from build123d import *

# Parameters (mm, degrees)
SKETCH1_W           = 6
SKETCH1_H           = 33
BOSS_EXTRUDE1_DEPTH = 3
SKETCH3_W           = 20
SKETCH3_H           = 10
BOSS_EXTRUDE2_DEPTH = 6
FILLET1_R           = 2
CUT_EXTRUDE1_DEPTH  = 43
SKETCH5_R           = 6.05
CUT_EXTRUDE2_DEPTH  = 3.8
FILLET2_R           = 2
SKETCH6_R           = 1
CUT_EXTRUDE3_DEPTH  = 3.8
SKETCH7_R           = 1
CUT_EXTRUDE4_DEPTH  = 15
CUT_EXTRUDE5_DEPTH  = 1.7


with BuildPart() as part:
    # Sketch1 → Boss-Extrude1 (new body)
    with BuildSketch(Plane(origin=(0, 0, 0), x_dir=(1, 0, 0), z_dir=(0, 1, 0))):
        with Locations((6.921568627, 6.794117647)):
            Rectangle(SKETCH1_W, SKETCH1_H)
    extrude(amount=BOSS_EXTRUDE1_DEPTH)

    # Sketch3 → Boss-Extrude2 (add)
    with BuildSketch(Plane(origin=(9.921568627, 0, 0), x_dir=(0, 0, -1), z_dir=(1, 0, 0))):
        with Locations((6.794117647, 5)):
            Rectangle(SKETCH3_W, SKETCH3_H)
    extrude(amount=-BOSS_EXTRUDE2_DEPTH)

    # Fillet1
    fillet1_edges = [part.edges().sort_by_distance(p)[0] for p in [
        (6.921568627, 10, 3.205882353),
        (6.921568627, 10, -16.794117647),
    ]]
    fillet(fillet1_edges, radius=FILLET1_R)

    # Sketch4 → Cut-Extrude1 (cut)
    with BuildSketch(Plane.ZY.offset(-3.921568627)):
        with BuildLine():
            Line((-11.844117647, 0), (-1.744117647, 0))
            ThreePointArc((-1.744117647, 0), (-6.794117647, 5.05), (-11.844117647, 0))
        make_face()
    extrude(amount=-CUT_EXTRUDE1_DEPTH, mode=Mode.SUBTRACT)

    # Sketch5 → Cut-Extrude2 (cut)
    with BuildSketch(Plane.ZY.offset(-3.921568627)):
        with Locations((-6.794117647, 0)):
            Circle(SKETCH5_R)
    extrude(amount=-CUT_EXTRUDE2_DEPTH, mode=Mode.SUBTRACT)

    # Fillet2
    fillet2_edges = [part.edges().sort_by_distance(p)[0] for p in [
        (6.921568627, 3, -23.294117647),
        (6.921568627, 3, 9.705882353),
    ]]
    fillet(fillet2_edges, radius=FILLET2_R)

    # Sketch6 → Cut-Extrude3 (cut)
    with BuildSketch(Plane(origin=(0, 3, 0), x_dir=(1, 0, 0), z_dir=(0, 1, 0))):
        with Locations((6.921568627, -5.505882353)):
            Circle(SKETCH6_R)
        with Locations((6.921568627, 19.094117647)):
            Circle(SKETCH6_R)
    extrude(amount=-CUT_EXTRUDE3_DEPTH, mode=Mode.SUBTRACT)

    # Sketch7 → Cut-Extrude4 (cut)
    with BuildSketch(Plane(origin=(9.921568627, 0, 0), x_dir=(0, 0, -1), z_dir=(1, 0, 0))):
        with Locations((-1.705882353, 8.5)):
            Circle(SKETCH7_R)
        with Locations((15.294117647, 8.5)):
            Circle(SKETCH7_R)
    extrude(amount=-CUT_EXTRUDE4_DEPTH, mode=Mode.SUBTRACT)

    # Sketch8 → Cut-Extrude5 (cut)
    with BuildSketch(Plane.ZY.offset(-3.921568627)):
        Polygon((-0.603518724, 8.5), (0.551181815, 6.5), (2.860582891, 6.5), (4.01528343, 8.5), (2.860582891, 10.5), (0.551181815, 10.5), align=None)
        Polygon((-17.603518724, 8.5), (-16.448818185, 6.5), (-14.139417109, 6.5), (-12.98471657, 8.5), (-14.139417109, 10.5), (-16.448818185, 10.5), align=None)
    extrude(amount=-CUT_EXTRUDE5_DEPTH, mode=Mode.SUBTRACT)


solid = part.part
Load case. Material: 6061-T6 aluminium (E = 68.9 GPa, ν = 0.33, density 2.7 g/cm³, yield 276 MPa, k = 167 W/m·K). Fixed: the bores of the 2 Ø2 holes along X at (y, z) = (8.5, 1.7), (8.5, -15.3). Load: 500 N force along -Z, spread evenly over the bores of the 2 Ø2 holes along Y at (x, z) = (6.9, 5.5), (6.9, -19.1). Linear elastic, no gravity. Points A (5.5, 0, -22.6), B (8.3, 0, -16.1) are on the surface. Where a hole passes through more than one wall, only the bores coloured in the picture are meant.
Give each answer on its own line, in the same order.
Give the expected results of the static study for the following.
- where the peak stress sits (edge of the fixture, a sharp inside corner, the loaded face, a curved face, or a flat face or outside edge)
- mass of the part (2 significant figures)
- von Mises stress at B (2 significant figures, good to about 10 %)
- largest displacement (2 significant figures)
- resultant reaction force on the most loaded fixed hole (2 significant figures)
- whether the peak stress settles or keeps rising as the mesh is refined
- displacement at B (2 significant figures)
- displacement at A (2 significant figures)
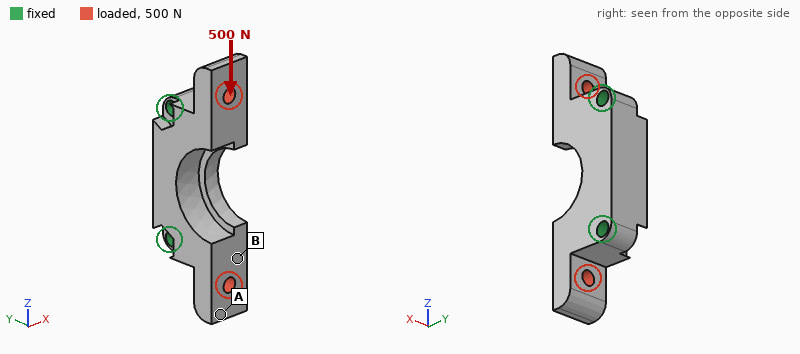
edge of the fixture
2.8 g
18 MPa
11 µm
300 N
keeps rising
6.4 µm
11 µm
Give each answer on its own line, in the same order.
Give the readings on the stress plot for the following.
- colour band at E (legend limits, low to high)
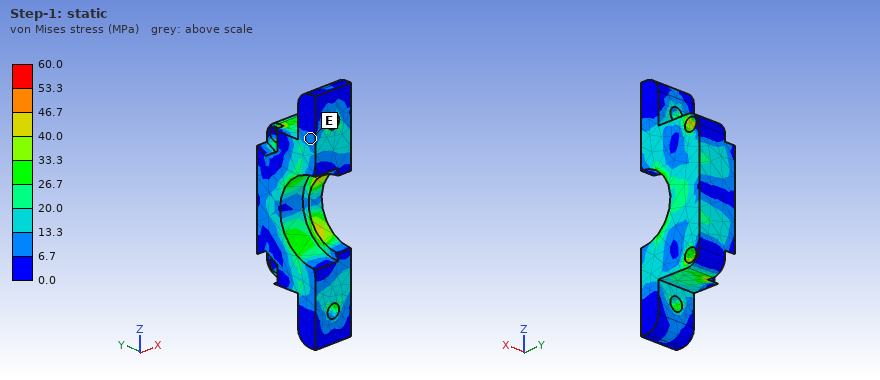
6.7 to 13.3 MPa
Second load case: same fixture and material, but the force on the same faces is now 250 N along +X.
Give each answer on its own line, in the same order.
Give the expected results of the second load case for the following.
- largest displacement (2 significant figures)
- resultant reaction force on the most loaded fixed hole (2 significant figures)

17 µm
130 N
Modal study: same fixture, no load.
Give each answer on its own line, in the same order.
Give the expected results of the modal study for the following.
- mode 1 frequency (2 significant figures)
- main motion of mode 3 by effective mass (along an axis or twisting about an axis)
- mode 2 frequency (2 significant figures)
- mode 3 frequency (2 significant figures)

24 kHz
twisting about Y
24 kHz
27 kHz
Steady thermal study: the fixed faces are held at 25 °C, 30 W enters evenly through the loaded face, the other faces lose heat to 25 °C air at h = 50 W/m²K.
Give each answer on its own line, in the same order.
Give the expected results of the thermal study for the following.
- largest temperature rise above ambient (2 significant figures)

43 K
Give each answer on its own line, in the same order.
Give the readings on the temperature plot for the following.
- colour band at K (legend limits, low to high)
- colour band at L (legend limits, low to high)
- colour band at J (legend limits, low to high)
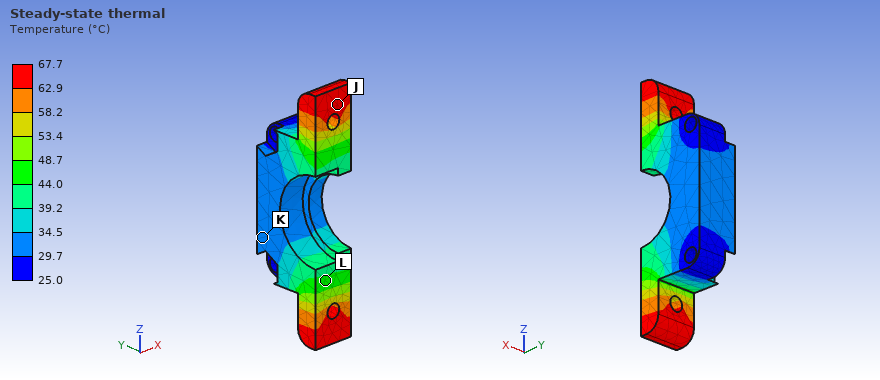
29.7 to 34.5 °C
44.0 to 48.7 °C
62.9 to 67.7 °C
